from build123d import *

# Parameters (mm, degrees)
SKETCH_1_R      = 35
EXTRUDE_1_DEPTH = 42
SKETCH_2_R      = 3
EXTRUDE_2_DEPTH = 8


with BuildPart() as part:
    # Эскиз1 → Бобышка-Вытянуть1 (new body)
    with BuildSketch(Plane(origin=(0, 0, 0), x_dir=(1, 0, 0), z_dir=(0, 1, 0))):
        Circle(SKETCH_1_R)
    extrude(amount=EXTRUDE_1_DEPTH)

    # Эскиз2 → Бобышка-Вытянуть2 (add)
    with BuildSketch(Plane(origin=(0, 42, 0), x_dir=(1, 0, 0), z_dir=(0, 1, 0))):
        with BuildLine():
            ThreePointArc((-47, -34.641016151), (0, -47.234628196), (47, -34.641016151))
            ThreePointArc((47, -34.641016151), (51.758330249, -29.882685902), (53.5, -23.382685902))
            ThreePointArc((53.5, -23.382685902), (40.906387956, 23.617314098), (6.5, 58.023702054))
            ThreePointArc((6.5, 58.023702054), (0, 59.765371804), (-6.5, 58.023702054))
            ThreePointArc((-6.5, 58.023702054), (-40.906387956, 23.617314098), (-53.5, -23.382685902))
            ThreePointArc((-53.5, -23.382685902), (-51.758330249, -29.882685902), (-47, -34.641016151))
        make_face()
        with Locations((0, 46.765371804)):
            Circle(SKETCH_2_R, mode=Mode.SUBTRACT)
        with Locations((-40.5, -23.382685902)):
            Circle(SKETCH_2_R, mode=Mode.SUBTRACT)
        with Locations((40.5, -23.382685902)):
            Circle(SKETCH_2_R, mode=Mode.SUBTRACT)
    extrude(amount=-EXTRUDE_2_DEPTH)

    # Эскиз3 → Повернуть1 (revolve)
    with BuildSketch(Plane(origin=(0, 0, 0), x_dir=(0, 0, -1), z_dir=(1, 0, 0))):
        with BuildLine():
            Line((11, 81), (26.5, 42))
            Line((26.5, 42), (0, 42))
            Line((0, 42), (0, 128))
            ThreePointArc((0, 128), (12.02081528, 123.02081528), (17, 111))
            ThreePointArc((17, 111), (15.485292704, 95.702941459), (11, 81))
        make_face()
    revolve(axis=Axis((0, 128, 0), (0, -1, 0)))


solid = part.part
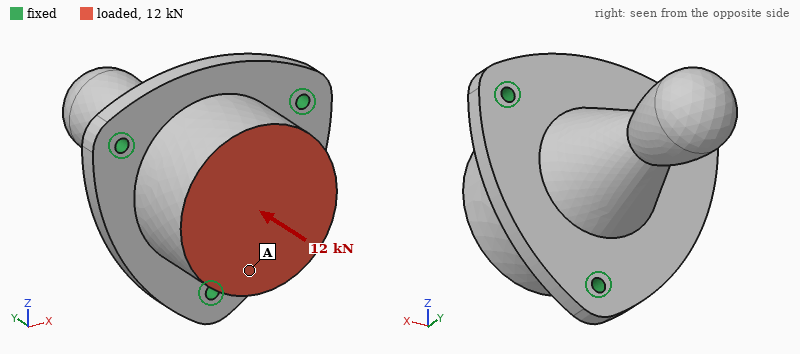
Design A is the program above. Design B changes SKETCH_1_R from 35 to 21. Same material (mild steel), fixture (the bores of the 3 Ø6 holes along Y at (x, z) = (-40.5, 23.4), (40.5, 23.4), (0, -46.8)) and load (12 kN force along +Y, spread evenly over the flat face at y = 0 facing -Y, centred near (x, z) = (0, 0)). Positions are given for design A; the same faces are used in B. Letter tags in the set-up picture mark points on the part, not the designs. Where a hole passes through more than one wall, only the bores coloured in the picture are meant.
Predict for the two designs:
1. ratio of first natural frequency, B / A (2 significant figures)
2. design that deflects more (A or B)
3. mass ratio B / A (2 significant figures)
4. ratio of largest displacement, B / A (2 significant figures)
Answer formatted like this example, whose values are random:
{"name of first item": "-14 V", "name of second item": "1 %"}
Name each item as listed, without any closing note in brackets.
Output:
{"ratio of first natural frequency, B / A": "0.82", "design that deflects more": "B", "mass ratio B / A": "0.70", "ratio of largest displacement, B / A": "2.3"}
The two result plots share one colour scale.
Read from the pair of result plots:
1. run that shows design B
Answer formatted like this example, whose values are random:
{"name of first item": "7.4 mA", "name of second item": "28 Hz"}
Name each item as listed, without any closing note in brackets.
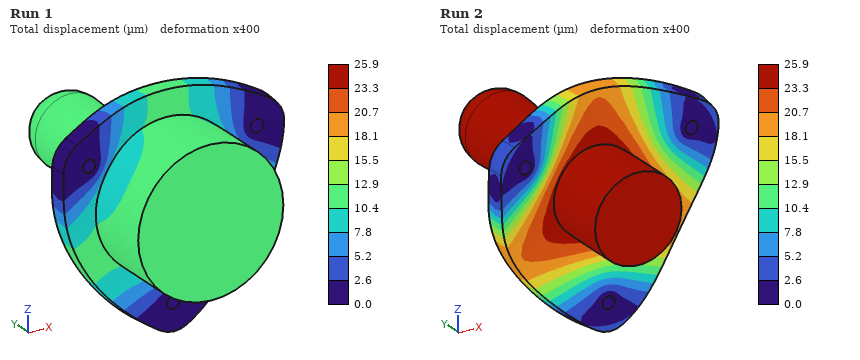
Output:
{"run that shows design B": "Run 2"}
